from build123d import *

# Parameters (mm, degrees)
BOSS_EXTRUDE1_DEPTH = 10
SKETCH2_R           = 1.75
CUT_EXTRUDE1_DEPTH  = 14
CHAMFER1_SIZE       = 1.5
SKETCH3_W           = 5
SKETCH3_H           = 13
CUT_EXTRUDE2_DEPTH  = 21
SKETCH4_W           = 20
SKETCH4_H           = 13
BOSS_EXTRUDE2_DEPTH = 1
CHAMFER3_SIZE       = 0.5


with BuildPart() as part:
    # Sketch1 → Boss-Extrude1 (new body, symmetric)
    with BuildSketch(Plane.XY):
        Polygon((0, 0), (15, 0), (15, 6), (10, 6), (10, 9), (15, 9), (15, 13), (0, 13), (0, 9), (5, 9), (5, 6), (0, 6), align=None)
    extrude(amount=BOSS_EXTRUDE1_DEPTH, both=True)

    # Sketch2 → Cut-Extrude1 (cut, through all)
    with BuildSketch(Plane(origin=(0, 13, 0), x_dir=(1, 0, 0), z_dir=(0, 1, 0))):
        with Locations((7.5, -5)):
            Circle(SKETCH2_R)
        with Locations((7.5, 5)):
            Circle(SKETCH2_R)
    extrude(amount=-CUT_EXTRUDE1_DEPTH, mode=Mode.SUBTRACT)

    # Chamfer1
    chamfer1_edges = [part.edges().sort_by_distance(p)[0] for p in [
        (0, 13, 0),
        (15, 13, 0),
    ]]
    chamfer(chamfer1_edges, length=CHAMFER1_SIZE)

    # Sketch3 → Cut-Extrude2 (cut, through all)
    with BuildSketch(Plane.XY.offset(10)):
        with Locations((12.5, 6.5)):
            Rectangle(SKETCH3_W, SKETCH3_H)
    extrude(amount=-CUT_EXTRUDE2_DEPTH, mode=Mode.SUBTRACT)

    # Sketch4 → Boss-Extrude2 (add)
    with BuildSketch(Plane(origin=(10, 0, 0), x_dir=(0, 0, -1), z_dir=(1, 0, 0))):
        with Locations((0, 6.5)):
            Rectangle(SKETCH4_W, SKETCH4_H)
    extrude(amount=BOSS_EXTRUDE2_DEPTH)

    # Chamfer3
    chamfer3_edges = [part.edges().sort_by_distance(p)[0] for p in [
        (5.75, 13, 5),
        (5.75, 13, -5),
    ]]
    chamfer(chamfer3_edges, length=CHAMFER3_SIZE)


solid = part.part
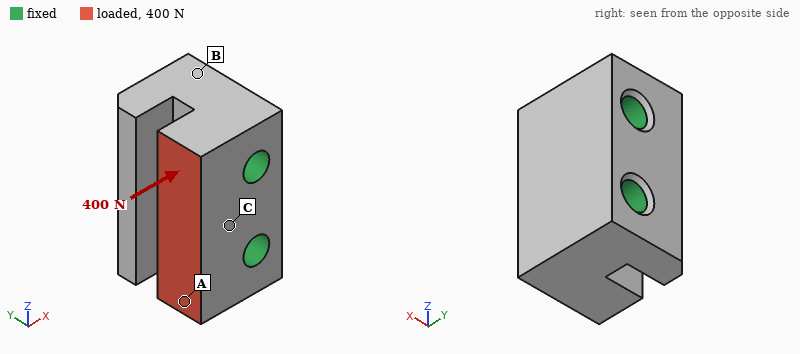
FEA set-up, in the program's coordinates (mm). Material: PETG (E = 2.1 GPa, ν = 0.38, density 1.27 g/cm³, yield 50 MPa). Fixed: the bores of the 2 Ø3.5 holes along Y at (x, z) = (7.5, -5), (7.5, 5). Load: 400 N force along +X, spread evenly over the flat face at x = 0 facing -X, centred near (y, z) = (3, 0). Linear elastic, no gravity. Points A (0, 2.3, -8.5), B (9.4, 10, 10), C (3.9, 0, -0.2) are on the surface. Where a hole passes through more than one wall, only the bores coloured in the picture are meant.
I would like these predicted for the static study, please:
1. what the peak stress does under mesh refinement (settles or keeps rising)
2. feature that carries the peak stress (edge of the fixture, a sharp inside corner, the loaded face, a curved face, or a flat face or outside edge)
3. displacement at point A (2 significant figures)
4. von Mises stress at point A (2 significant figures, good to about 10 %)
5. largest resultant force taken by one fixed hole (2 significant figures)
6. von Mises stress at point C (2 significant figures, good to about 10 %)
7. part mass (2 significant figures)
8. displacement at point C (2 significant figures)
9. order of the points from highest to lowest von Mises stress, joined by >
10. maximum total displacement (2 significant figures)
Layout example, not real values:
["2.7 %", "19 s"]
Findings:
["keeps rising", "edge of the fixture", "16 µm", "3.4 MPa", "200 N", "1.9 MPa", "2.9 g", "7.3 µm", "A > C > B", "19 µm"]
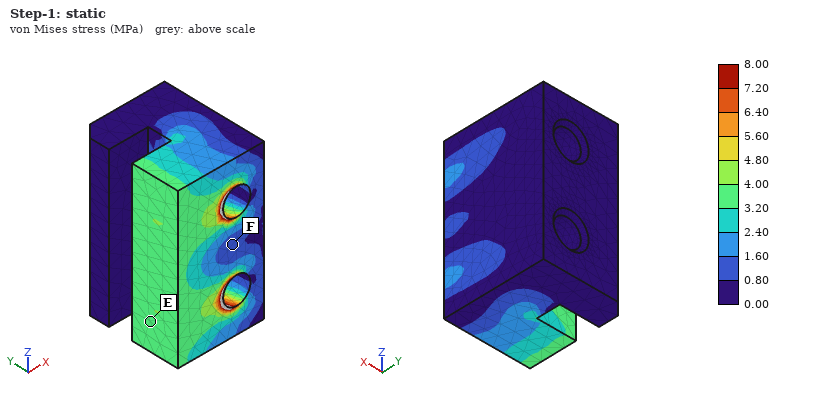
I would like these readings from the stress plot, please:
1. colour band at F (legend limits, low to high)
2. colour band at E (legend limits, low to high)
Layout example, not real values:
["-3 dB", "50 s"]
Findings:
["0.80 to 1.60 MPa", "3.20 to 4.00 MPa"]
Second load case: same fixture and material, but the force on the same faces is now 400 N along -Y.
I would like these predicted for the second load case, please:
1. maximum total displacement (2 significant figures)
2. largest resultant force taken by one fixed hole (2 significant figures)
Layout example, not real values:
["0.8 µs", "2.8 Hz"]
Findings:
["89 µm", "200 N"]
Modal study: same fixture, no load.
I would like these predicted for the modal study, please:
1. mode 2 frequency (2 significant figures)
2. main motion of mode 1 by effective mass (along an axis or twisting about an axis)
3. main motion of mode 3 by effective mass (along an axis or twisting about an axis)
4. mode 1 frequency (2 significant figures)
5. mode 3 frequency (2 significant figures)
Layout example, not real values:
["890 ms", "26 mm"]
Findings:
["19 kHz", "along Y", "along Y", "18 kHz", "20 kHz"]
